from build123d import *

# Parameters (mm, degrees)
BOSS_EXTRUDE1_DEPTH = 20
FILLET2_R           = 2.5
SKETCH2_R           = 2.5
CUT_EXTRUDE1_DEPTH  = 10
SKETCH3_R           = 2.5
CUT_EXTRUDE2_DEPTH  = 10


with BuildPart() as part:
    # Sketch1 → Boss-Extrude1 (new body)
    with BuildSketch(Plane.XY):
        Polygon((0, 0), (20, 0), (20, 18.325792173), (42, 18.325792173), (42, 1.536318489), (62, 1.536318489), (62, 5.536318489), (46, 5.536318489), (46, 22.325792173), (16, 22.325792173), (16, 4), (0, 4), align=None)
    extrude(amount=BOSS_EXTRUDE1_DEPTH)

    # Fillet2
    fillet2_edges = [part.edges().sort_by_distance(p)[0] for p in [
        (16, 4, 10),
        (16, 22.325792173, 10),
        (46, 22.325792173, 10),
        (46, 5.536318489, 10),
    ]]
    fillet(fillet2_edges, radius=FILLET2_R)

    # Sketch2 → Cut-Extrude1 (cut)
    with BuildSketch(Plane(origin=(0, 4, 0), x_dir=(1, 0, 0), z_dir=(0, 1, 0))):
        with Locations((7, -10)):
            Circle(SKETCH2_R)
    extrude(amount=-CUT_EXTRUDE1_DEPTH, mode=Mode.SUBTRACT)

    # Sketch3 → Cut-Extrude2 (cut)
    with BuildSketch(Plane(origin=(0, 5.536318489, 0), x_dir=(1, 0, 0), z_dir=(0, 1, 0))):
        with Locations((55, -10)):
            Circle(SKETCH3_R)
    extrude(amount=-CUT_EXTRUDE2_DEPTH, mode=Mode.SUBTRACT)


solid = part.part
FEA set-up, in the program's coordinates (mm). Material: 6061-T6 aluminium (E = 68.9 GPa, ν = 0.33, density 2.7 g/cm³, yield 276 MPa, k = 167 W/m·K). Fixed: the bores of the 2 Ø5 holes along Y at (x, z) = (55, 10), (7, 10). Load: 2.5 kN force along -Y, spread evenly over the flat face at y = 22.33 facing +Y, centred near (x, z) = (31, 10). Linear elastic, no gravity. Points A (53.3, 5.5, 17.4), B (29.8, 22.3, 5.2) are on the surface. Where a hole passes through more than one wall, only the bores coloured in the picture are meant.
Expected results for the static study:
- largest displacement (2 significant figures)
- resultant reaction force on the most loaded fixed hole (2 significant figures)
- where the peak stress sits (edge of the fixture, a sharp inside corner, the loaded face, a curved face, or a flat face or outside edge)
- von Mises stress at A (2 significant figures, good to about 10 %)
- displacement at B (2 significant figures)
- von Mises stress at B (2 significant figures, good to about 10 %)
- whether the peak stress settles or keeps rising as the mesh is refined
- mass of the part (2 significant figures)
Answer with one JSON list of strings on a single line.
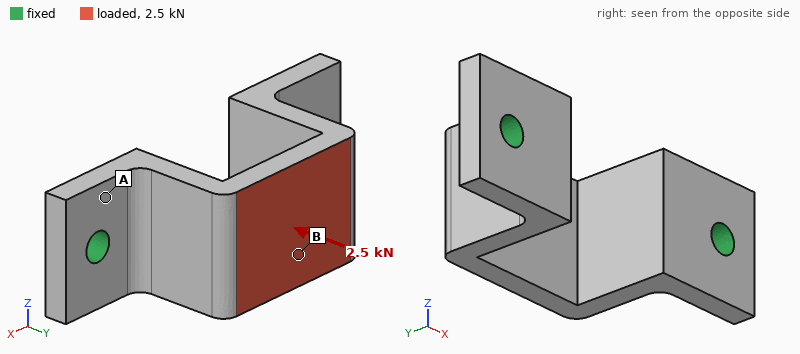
["55 µm", "1.4 kN", "edge of the fixture", "29 MPa", "51 µm", "60 MPa", "keeps rising", "21 g"]
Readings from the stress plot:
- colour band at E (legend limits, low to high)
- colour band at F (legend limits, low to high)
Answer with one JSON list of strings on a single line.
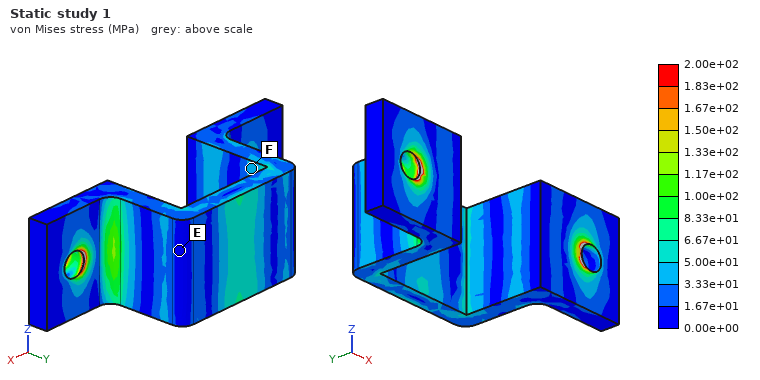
["0.00e+00 to 1.67e+01 MPa", "3.33e+01 to 5.00e+01 MPa"]
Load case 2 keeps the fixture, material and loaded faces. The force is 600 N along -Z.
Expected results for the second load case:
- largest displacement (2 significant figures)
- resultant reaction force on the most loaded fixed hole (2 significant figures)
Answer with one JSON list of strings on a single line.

["97 µm", "310 N"]
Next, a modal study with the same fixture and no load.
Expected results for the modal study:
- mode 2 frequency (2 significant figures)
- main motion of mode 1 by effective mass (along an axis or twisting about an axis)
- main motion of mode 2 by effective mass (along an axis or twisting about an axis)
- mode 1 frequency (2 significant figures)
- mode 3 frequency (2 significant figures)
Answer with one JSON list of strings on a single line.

["7100 Hz", "along Z", "along X", "4800 Hz", "9300 Hz"]
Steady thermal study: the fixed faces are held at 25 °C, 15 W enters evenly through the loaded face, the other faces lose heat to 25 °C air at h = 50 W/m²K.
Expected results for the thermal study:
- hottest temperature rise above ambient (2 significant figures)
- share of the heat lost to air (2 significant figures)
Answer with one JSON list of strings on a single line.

["17 K", "9.7 %"]
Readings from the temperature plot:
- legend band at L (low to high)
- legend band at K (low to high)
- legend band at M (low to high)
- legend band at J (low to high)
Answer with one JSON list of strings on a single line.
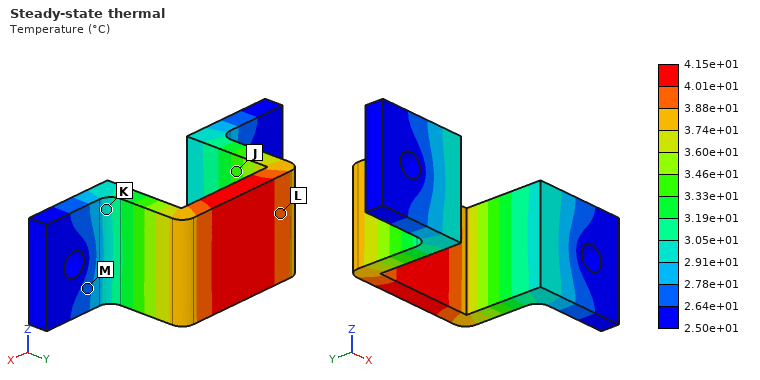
["3.88e+01 to 4.01e+01 °C", "2.91e+01 to 3.05e+01 °C", "2.64e+01 to 2.78e+01 °C", "3.33e+01 to 3.46e+01 °C"]
